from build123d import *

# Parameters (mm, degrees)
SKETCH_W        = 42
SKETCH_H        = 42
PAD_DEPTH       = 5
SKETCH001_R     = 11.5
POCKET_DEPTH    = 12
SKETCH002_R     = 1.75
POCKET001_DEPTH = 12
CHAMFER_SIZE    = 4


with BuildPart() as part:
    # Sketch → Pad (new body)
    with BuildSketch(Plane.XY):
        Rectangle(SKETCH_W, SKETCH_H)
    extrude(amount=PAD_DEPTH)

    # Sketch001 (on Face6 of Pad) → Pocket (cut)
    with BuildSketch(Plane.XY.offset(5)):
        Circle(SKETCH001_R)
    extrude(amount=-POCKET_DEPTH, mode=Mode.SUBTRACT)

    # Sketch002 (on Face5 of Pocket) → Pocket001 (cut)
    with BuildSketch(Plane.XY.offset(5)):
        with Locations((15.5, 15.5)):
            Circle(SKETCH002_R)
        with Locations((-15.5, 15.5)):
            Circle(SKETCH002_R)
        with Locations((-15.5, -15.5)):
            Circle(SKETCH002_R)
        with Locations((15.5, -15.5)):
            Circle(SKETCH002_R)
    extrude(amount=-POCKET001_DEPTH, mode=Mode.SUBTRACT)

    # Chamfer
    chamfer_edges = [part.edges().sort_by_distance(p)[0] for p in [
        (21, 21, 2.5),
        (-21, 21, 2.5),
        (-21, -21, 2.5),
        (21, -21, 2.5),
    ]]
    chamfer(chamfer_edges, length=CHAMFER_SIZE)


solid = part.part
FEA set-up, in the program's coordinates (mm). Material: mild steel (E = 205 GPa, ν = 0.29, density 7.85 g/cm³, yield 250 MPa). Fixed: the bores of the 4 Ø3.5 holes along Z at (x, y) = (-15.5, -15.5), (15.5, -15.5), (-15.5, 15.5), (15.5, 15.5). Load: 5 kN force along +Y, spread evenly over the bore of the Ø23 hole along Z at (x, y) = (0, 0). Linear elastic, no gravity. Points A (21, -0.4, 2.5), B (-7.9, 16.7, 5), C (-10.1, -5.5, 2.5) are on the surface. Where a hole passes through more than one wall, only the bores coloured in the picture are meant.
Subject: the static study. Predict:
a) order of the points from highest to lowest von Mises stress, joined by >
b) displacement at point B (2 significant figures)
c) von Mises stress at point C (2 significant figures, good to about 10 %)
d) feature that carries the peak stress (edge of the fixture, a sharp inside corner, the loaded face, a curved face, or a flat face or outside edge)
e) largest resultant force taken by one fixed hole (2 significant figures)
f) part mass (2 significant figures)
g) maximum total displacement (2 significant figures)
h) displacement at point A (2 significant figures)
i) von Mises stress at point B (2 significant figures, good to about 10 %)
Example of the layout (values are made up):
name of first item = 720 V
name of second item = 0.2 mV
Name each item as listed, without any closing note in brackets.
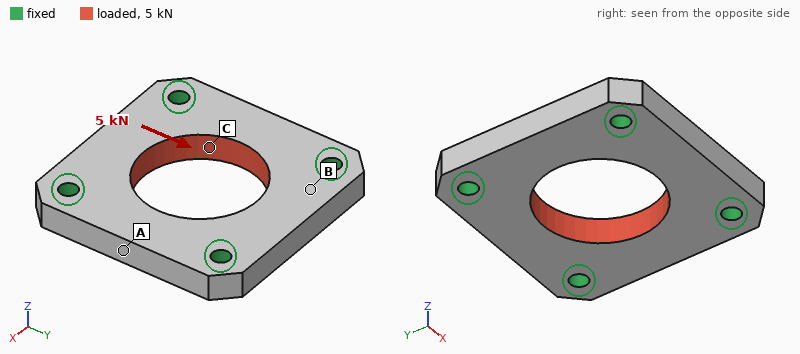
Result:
order of the points from highest to lowest von Mises stress, joined by > = C > B > A
displacement at point B = 1.8 µm
von Mises stress at point C = 31 MPa
feature that carries the peak stress = edge of the fixture
largest resultant force taken by one fixed hole = 1.3 kN
part mass = 50 g
maximum total displacement = 3.1 µm
displacement at point A = 0.77 µm
von Mises stress at point B = 18 MPa
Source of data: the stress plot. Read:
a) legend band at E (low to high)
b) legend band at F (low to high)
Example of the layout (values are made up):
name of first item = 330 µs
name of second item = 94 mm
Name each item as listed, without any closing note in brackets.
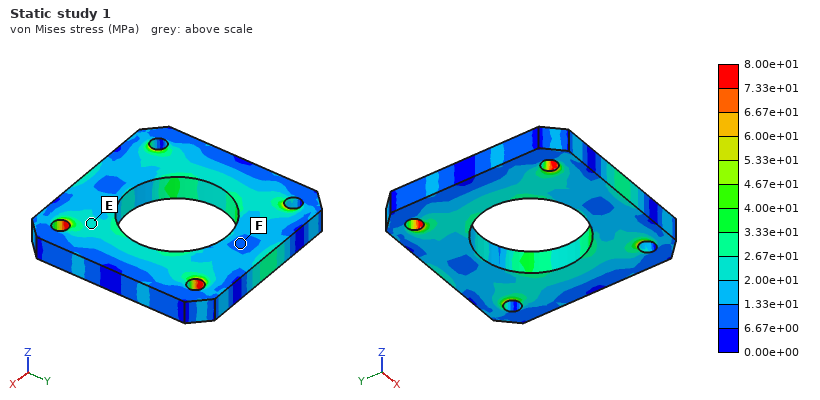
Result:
legend band at E = 2.00e+01 to 2.67e+01 MPa
legend band at F = 6.67e+00 to 1.33e+01 MPa
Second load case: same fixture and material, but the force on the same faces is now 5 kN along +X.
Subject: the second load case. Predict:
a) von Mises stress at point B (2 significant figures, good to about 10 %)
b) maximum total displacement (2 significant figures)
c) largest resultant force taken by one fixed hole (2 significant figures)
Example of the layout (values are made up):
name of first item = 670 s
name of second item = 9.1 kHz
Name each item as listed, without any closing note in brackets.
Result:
von Mises stress at point B = 16 MPa
maximum total displacement = 3.1 µm
largest resultant force taken by one fixed hole = 1.3 kN
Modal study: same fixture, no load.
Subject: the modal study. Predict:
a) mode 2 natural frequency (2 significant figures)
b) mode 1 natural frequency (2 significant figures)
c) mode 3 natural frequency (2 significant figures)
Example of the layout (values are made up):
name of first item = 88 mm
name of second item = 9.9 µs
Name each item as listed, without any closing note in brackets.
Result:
mode 2 natural frequency = 25 kHz
mode 1 natural frequency = 25 kHz
mode 3 natural frequency = 26 kHz
